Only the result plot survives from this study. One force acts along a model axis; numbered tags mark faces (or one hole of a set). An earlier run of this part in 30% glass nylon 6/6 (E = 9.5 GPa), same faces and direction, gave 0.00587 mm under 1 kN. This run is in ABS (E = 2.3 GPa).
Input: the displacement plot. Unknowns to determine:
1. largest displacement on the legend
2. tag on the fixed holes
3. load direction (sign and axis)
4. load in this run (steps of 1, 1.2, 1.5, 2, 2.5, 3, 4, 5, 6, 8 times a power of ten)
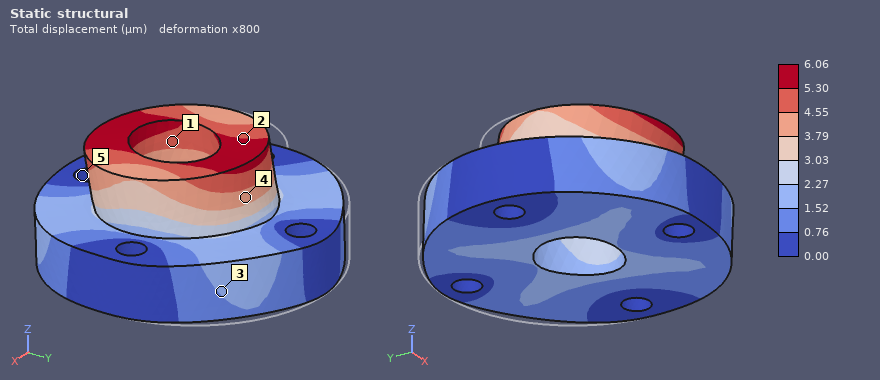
6.06 µm
5
-Y
250 N
